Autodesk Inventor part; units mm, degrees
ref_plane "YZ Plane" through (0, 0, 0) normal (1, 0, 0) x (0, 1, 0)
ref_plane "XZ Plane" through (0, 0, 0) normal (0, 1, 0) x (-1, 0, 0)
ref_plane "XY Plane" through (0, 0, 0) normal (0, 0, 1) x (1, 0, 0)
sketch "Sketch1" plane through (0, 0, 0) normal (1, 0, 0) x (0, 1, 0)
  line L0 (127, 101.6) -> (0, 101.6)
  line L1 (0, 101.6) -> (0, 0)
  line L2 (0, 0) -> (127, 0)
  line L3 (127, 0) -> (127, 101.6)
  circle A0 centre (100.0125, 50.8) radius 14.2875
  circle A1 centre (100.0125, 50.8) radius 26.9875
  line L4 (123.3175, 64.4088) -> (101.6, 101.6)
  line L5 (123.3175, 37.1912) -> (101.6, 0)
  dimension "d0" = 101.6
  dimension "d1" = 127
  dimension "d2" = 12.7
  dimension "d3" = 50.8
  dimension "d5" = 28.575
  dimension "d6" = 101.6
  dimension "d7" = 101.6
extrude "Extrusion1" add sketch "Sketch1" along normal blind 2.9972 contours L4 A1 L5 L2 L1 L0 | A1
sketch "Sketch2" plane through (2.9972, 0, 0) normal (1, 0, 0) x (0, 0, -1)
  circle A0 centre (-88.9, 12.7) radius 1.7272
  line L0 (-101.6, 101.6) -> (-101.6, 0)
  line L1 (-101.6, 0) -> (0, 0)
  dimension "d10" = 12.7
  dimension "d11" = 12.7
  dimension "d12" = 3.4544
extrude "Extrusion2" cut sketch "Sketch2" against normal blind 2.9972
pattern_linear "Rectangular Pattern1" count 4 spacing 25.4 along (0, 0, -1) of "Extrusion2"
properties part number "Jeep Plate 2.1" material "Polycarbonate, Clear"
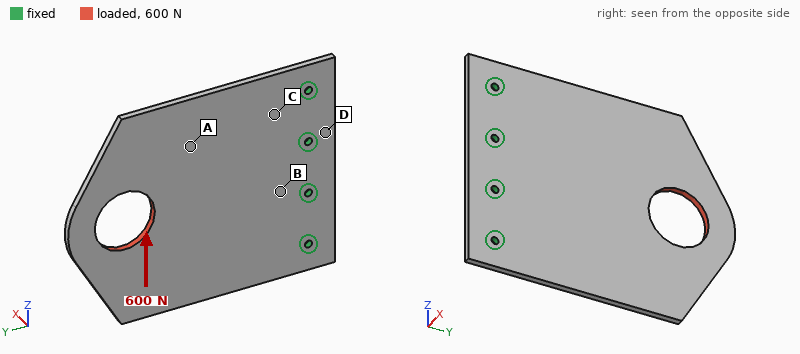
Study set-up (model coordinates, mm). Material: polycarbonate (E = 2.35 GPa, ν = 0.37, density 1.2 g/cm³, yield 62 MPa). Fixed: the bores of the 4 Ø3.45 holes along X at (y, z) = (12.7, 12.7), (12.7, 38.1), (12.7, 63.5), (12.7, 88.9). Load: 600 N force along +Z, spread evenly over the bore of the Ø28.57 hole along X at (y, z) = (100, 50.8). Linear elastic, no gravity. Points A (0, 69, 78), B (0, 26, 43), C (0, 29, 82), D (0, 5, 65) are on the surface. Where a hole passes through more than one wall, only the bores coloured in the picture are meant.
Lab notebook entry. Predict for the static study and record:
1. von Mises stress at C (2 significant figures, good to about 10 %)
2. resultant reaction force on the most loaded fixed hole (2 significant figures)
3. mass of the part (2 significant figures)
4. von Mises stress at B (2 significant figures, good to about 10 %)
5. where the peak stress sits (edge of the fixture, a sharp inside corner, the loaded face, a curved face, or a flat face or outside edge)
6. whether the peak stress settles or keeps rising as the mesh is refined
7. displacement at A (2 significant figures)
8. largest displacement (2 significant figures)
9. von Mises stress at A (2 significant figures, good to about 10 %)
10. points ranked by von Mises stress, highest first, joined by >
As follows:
7.1 MPa
650 N
40 g
5.2 MPa
edge of the fixture
keeps rising
0.33 mm
0.72 mm
3.4 MPa
C > B > A > D
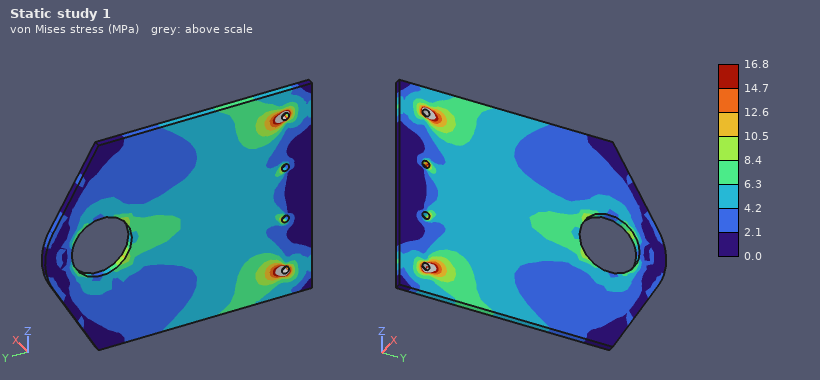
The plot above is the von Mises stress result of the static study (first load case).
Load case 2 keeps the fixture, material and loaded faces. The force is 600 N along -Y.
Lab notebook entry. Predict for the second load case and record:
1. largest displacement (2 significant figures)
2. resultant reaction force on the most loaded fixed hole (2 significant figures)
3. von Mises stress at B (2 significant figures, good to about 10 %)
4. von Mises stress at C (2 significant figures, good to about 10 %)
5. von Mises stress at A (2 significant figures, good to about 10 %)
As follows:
0.17 mm
160 N
2.0 MPa
2.1 MPa
2.4 MPa
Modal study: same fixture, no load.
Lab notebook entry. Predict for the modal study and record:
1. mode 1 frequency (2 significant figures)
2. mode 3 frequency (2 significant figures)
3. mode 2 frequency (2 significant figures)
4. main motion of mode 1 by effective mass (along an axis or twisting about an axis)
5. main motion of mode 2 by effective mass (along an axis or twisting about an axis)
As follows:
69 Hz
350 Hz
170 Hz
along X
twisting about Y
